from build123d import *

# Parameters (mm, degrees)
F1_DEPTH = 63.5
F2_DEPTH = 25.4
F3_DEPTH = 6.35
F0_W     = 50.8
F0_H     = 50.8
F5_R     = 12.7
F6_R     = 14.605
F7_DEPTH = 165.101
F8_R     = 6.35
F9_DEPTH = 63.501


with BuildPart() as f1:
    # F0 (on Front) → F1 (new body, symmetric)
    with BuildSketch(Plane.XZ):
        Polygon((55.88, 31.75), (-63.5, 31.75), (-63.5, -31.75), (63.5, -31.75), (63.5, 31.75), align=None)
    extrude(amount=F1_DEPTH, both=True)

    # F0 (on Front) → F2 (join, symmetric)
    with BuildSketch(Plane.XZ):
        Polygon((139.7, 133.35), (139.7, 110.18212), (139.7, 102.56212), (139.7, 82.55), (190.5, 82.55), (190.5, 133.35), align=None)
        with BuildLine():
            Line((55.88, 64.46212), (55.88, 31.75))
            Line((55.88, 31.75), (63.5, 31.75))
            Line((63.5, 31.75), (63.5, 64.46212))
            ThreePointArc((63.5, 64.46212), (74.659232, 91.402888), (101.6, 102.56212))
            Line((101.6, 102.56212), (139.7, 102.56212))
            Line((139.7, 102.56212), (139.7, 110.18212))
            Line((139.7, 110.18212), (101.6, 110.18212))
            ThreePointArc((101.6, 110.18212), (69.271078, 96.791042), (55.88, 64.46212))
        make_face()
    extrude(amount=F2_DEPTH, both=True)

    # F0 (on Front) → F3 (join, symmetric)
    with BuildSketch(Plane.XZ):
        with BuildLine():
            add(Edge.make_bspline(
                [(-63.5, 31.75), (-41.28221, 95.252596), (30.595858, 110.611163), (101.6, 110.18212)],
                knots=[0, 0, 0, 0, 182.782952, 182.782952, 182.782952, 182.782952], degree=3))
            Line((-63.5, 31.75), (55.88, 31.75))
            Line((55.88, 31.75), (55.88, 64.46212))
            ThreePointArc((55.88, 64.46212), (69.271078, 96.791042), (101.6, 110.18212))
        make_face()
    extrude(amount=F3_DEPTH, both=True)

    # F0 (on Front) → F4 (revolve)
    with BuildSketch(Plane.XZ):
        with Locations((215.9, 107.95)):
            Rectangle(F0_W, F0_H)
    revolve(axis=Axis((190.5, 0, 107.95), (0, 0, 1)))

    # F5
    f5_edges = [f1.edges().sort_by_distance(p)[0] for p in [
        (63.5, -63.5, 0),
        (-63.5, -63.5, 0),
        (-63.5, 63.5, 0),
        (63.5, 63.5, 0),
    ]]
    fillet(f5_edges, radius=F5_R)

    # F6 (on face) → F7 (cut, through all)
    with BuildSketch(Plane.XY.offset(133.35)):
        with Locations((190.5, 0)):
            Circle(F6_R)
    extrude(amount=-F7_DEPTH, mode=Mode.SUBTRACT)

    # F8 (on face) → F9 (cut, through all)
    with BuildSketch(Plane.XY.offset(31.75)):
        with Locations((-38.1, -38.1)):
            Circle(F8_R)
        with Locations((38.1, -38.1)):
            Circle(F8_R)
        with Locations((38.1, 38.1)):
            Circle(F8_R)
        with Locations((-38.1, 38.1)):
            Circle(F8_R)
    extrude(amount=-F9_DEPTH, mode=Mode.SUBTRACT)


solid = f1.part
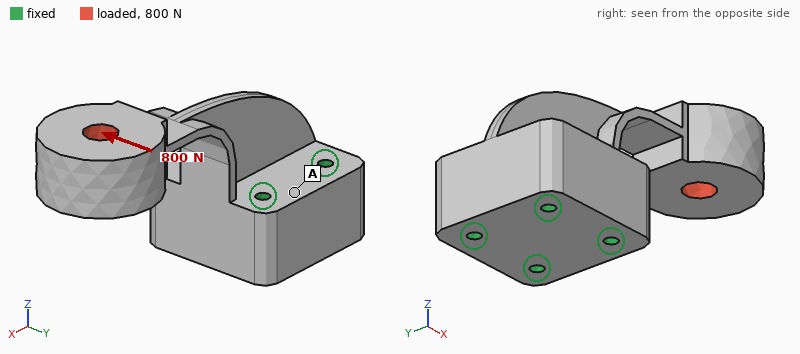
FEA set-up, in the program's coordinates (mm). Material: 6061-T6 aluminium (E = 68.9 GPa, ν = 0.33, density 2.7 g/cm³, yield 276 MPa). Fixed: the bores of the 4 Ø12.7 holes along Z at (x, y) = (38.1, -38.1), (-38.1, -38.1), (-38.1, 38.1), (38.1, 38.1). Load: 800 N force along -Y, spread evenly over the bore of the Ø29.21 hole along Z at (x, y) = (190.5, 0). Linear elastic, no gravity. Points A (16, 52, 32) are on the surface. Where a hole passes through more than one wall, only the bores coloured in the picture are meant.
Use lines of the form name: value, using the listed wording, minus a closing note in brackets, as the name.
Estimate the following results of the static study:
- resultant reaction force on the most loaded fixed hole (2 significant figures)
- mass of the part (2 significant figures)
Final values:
resultant reaction force on the most loaded fixed hole: 1.8 kN
mass of the part: 4.1 kg
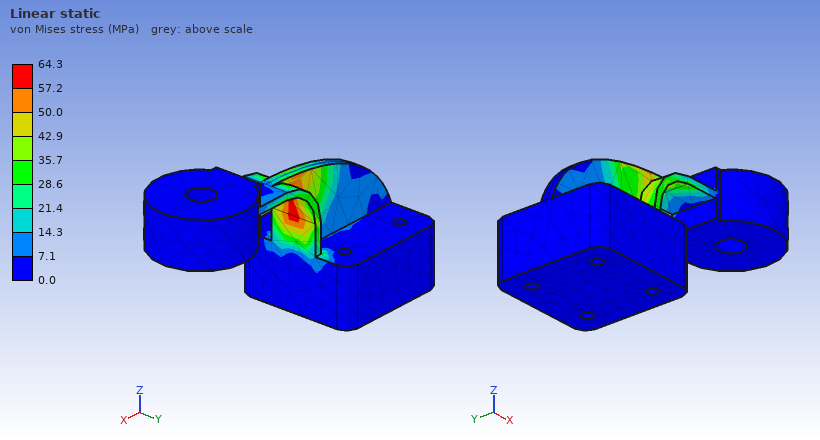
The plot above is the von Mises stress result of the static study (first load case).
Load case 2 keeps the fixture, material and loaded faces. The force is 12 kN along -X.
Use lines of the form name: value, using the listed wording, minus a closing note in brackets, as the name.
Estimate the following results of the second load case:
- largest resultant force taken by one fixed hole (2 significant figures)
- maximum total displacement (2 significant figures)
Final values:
largest resultant force taken by one fixed hole: 7.0 kN
maximum total displacement: 2.3 mm
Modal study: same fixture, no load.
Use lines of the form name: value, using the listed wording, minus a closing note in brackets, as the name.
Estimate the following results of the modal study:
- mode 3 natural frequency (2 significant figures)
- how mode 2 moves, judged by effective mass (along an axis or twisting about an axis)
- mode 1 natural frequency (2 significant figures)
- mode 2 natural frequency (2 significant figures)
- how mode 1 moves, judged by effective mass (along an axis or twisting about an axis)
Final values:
mode 3 natural frequency: 330 Hz
how mode 2 moves, judged by effective mass: along Y
mode 1 natural frequency: 83 Hz
mode 2 natural frequency: 130 Hz
how mode 1 moves, judged by effective mass: along Z
